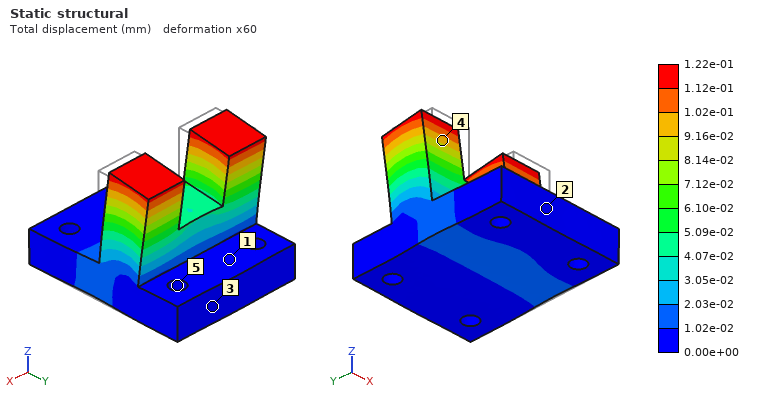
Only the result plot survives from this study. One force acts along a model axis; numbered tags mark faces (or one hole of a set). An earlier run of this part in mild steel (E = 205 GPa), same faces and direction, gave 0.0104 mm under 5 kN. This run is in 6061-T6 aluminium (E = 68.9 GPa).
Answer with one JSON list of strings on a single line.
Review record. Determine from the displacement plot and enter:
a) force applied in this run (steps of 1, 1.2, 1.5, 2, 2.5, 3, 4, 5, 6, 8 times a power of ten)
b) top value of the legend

["20 kN", "1.22e-01 mm"]
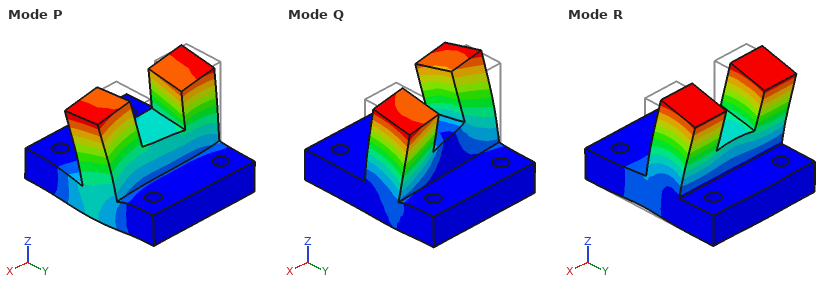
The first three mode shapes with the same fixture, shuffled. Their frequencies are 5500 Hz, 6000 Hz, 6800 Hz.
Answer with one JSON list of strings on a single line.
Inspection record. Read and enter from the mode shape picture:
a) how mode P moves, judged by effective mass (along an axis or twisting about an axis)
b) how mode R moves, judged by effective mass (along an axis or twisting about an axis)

["along X", "along Y"]
